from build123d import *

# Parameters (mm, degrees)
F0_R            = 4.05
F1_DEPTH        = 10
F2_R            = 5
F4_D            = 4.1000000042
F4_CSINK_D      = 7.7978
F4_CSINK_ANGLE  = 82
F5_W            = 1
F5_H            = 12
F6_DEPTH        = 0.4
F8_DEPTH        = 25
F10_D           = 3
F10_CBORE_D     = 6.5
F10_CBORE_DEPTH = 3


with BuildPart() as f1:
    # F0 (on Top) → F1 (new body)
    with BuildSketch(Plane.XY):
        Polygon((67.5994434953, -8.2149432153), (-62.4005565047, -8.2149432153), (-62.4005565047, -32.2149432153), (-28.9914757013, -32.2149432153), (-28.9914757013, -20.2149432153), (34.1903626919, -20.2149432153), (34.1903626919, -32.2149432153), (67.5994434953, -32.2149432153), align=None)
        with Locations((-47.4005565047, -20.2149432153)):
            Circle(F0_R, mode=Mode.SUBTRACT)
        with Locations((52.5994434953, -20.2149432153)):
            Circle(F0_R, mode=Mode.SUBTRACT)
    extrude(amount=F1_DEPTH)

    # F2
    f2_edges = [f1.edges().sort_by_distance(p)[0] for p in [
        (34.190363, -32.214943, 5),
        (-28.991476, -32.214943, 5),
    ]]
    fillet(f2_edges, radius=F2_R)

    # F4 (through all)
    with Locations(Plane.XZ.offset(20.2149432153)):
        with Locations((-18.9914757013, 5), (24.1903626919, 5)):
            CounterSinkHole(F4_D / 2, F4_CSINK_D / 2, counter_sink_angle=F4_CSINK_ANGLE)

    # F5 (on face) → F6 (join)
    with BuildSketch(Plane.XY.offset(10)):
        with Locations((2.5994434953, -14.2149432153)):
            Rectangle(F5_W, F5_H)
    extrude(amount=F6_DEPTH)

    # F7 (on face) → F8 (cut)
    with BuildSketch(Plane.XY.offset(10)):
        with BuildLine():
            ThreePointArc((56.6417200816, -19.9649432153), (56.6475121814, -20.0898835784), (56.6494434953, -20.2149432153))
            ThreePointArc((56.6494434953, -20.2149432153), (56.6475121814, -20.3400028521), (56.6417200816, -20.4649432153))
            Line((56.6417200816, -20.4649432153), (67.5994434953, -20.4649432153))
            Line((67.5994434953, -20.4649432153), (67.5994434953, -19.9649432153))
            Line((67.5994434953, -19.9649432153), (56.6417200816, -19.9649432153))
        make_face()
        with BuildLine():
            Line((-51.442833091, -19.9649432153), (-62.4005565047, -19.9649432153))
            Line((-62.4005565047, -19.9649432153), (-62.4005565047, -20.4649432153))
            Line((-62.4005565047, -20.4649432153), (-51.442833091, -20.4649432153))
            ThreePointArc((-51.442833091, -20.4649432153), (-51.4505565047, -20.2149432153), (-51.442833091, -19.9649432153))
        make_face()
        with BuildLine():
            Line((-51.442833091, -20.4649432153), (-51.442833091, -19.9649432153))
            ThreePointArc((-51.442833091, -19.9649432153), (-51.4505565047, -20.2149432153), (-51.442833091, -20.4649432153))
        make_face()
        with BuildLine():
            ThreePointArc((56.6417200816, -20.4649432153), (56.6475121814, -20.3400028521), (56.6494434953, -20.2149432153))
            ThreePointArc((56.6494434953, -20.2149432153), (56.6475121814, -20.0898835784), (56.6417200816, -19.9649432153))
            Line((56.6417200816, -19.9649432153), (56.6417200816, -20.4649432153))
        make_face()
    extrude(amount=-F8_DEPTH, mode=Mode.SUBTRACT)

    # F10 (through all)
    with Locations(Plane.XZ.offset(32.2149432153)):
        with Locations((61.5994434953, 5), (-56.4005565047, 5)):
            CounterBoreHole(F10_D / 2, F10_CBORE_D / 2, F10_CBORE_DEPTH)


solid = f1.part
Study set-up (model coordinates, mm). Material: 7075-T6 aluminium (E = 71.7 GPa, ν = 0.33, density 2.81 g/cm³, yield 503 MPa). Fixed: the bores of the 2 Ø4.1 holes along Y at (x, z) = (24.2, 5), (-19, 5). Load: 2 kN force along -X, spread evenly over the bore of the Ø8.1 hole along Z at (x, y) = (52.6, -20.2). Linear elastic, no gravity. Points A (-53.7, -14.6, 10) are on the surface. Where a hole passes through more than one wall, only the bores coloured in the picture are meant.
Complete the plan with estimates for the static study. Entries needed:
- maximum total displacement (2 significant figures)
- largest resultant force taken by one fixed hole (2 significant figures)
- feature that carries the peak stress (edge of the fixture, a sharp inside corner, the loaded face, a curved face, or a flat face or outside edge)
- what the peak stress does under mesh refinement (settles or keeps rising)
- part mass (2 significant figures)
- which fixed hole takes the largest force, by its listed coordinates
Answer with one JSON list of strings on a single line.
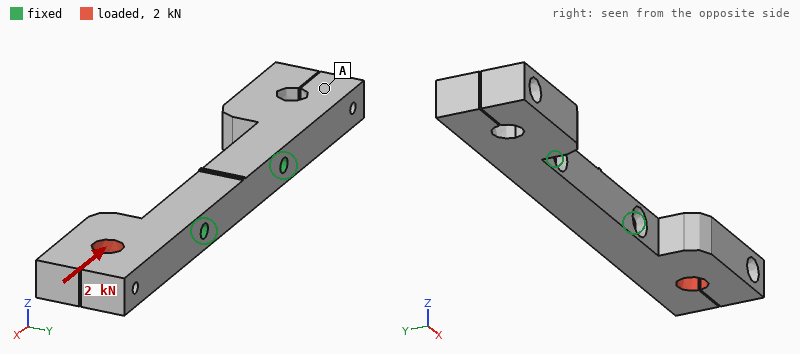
["87 µm", "1.9 kN", "edge of the fixture", "keeps rising", "60 g", "(24.2, 5)"]
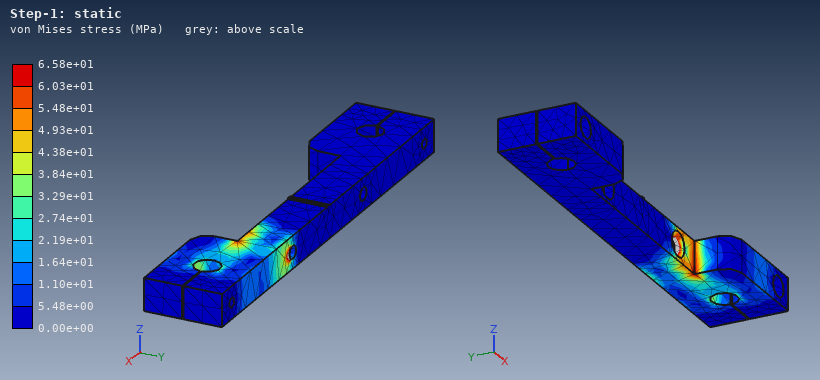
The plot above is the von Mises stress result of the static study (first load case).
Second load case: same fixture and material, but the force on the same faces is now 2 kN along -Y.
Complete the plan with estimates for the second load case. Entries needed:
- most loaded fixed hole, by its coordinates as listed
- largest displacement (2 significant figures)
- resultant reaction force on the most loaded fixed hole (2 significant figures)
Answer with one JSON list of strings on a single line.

["(24.2, 5)", "0.32 mm", "2.1 kN"]
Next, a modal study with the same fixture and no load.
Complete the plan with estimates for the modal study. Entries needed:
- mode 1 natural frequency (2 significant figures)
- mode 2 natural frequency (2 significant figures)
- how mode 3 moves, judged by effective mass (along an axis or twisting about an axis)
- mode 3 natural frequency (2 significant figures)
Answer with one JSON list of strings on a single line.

["2900 Hz", "2900 Hz", "along Y", "3500 Hz"]
